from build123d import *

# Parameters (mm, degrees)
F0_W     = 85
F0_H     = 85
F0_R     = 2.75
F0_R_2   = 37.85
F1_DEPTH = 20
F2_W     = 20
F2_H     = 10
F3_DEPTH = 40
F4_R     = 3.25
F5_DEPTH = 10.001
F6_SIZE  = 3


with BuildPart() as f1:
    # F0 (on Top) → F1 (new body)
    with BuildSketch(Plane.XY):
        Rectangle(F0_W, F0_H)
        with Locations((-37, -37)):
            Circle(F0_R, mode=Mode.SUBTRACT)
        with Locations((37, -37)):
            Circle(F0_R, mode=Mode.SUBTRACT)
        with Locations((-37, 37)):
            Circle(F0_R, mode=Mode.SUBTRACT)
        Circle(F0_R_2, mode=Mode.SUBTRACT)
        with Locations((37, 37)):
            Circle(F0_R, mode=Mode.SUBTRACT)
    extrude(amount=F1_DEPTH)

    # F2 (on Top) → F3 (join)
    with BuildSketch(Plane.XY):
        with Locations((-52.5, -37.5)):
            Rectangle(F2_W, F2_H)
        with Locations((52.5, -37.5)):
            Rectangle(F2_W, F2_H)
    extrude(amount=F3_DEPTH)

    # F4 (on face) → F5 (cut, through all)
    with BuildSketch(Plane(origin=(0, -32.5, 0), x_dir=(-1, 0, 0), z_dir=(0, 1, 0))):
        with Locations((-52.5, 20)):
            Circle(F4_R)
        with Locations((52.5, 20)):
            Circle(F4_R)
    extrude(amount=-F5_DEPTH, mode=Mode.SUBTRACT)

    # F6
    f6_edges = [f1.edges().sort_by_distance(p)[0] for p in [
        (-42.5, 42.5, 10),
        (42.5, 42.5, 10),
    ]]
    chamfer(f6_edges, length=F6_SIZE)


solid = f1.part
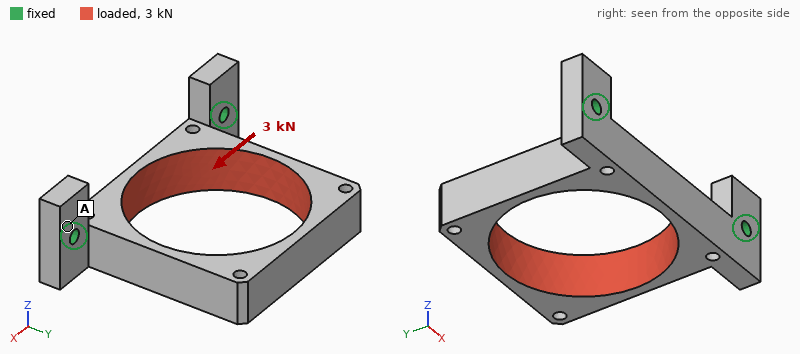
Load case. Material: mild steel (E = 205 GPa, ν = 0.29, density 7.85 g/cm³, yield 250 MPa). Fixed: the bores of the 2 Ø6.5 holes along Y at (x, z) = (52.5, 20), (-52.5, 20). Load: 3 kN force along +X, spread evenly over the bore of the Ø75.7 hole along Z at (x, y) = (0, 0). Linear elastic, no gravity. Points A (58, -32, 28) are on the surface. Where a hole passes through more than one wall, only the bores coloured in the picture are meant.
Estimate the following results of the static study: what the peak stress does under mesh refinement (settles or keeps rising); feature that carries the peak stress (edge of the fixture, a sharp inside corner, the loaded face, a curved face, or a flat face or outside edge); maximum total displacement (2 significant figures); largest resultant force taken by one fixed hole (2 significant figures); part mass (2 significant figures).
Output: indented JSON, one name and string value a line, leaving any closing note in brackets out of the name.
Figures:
{
  "what the peak stress does under mesh refinement": "keeps rising",
  "feature that carries the peak stress": "a sharp inside corner",
  "maximum total displacement": "94 µm",
  "largest resultant force taken by one fixed hole": "1.8 kN",
  "part mass": "530 g"
}
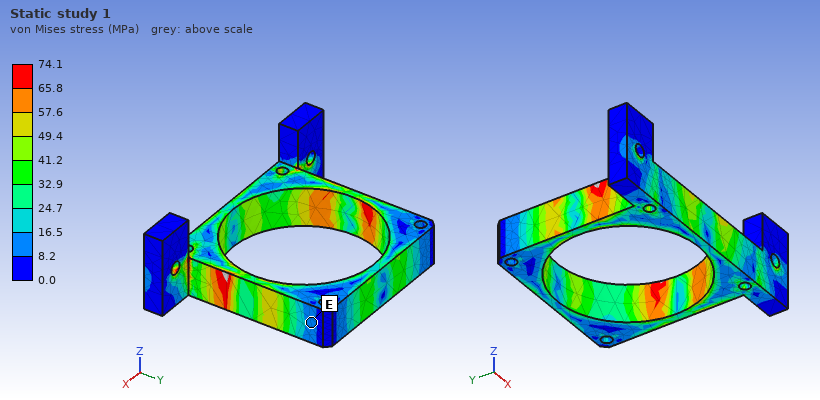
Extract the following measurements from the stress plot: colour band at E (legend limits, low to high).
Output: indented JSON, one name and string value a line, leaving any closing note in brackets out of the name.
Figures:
{
  "colour band at E": "8.2 to 16.5 MPa"
}
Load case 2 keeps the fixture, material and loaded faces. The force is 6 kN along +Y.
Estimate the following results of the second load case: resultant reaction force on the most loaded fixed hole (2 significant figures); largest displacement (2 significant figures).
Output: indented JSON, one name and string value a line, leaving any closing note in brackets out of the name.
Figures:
{
  "resultant reaction force on the most loaded fixed hole": "3.0 kN",
  "largest displacement": "60 µm"
}
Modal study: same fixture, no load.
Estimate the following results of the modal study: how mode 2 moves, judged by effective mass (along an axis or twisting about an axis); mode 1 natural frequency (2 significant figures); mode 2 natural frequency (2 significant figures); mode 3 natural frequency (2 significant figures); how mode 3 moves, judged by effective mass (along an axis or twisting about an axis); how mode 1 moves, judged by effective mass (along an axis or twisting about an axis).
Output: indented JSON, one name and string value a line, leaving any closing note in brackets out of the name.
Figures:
{
  "how mode 2 moves, judged by effective mass": "along X",
  "mode 1 natural frequency": "940 Hz",
  "mode 2 natural frequency": "1500 Hz",
  "mode 3 natural frequency": "1800 Hz",
  "how mode 3 moves, judged by effective mass": "twisting about Y",
  "how mode 1 moves, judged by effective mass": "along Z"
}
